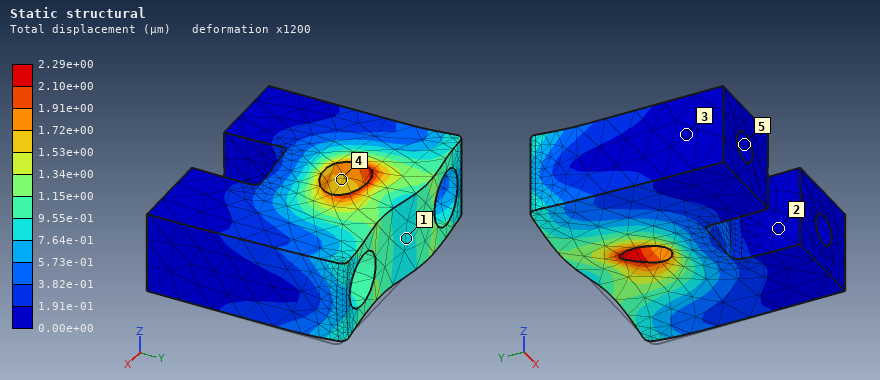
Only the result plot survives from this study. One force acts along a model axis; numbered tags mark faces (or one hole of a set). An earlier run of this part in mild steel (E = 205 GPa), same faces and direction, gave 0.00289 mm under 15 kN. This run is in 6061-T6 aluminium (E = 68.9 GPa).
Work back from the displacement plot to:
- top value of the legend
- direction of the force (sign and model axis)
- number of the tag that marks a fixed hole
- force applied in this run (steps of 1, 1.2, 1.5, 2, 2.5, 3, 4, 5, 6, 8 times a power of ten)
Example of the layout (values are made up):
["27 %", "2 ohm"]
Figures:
["2.29e+00 µm", "-X", "5", "4 kN"]
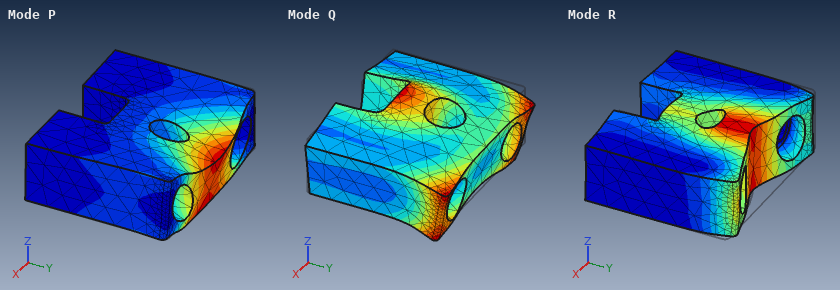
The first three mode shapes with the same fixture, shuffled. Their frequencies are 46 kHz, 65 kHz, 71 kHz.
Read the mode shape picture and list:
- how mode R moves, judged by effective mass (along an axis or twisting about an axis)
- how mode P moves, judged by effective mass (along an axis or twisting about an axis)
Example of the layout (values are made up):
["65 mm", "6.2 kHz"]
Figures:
["along Y", "along Z"]
